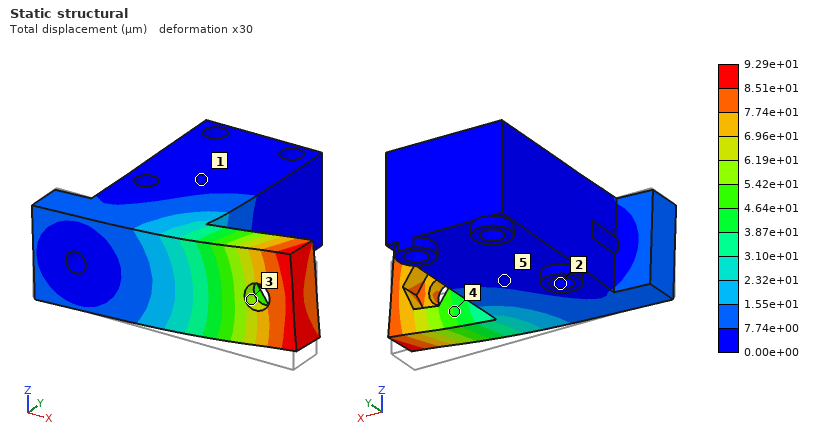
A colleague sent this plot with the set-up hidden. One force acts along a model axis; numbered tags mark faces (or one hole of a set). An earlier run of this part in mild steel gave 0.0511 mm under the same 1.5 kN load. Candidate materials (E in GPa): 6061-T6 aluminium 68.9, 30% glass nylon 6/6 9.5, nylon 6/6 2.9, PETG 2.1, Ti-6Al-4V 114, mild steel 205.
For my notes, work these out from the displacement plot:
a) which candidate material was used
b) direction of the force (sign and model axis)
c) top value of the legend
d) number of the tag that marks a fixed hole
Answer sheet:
Ti-6Al-4V
+Z
9.29e+01 µm
2
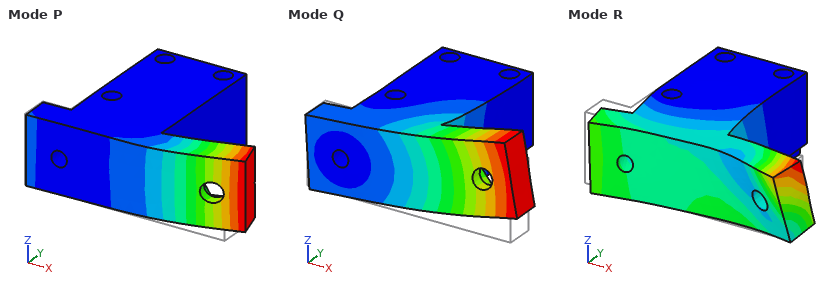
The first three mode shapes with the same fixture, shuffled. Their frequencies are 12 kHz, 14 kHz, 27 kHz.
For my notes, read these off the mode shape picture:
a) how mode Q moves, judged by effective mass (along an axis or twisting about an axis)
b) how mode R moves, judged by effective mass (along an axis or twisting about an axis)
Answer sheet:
along Z
along X
